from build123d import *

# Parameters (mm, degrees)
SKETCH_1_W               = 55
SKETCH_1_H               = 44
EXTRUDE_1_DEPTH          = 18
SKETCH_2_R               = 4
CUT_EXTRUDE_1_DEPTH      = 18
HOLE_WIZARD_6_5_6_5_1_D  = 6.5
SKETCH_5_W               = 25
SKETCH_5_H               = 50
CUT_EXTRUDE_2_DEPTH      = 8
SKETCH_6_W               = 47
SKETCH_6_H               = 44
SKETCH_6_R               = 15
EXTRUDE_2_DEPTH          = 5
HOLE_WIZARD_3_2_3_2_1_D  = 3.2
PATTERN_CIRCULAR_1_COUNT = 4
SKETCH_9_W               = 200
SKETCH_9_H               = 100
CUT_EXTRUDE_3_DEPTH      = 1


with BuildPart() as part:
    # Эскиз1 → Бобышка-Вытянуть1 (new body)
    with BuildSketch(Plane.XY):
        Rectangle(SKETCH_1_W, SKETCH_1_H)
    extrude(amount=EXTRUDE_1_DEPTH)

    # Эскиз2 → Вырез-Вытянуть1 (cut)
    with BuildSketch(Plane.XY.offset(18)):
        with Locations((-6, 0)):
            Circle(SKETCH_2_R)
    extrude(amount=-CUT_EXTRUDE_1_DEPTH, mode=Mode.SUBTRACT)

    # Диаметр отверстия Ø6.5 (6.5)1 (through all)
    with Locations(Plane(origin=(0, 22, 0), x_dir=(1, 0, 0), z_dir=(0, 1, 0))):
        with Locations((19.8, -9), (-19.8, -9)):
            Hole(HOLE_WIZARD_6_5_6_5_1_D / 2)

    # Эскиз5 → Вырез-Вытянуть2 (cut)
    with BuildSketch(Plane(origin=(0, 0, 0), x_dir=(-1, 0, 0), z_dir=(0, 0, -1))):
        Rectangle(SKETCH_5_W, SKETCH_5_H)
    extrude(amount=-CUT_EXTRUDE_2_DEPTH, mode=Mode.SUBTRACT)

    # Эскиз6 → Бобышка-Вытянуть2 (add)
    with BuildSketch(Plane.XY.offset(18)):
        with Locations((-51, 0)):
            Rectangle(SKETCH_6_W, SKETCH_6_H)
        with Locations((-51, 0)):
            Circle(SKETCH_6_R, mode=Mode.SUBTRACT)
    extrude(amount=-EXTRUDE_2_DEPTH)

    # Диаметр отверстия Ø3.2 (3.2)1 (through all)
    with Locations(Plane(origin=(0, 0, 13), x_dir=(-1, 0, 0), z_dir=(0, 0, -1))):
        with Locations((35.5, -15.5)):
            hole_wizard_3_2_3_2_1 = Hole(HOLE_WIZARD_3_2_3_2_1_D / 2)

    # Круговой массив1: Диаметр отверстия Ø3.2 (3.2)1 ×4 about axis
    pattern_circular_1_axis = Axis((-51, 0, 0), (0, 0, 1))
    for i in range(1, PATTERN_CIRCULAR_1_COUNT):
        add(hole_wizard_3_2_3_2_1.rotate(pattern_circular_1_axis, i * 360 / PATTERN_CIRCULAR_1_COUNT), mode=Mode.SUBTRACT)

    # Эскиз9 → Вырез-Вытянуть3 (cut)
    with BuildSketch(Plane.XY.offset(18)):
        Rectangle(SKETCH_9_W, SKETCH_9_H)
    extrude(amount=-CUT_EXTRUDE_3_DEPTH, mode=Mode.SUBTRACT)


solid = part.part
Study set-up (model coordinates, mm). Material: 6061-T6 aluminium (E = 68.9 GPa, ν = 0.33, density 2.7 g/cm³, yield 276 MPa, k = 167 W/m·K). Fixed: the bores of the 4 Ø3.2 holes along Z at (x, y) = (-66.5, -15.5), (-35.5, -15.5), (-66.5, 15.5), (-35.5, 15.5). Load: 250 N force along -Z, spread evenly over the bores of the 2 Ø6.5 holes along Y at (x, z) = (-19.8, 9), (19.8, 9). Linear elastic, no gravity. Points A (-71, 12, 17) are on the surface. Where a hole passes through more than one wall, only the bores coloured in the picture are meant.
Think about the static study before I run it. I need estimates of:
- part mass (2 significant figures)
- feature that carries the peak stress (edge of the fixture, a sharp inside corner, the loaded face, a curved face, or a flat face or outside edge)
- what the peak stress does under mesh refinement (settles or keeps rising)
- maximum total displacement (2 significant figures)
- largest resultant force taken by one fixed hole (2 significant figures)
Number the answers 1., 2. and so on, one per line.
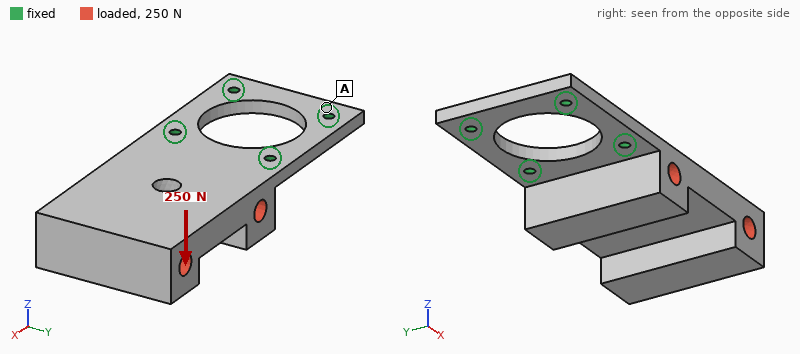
1. 93 g
2. edge of the fixture
3. keeps rising
4. 0.38 mm
5. 140 N
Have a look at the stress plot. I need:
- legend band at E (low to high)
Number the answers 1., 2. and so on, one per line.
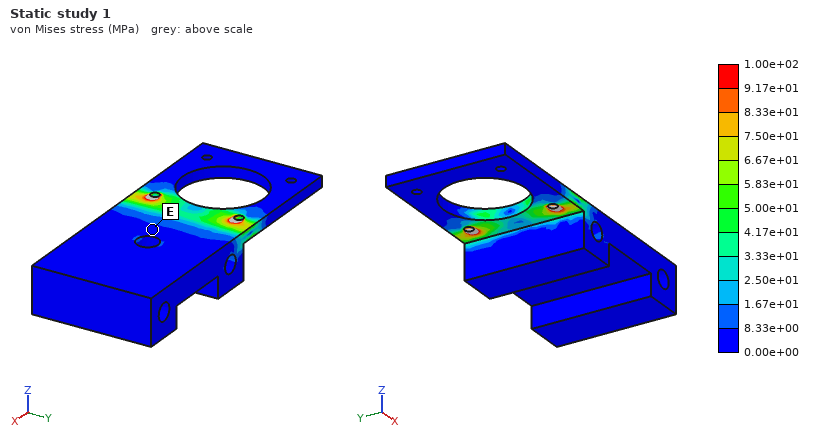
1. 0.00e+00 to 8.33e+00 MPa
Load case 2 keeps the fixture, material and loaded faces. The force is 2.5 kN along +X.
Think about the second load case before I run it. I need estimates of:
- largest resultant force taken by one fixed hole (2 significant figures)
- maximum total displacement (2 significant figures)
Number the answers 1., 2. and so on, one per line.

1. 1.2 kN
2. 0.71 mm
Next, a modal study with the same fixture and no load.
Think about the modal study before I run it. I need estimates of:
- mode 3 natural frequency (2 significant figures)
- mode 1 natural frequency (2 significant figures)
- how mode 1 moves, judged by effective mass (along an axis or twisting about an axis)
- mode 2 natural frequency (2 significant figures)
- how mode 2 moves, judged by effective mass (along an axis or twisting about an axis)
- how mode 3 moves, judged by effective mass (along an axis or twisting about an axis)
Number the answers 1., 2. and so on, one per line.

1. 4300 Hz
2. 550 Hz
3. along Z
4. 3900 Hz
5. along Y
6. along Y
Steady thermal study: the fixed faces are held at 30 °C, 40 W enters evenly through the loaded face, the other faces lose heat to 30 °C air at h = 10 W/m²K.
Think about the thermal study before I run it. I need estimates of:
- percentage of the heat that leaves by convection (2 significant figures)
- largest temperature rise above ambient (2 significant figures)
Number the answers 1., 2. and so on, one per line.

1. 6.0 %
2. 34 K
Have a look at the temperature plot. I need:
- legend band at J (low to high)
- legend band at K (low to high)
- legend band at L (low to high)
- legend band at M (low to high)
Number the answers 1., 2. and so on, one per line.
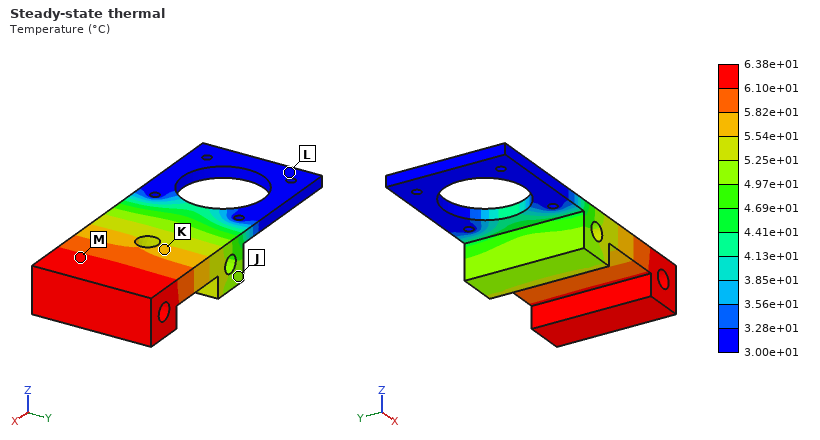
1. 4.97e+01 to 5.25e+01 °C
2. 5.54e+01 to 5.82e+01 °C
3. 3.00e+01 to 3.28e+01 °C
4. 6.10e+01 to 6.38e+01 °C
